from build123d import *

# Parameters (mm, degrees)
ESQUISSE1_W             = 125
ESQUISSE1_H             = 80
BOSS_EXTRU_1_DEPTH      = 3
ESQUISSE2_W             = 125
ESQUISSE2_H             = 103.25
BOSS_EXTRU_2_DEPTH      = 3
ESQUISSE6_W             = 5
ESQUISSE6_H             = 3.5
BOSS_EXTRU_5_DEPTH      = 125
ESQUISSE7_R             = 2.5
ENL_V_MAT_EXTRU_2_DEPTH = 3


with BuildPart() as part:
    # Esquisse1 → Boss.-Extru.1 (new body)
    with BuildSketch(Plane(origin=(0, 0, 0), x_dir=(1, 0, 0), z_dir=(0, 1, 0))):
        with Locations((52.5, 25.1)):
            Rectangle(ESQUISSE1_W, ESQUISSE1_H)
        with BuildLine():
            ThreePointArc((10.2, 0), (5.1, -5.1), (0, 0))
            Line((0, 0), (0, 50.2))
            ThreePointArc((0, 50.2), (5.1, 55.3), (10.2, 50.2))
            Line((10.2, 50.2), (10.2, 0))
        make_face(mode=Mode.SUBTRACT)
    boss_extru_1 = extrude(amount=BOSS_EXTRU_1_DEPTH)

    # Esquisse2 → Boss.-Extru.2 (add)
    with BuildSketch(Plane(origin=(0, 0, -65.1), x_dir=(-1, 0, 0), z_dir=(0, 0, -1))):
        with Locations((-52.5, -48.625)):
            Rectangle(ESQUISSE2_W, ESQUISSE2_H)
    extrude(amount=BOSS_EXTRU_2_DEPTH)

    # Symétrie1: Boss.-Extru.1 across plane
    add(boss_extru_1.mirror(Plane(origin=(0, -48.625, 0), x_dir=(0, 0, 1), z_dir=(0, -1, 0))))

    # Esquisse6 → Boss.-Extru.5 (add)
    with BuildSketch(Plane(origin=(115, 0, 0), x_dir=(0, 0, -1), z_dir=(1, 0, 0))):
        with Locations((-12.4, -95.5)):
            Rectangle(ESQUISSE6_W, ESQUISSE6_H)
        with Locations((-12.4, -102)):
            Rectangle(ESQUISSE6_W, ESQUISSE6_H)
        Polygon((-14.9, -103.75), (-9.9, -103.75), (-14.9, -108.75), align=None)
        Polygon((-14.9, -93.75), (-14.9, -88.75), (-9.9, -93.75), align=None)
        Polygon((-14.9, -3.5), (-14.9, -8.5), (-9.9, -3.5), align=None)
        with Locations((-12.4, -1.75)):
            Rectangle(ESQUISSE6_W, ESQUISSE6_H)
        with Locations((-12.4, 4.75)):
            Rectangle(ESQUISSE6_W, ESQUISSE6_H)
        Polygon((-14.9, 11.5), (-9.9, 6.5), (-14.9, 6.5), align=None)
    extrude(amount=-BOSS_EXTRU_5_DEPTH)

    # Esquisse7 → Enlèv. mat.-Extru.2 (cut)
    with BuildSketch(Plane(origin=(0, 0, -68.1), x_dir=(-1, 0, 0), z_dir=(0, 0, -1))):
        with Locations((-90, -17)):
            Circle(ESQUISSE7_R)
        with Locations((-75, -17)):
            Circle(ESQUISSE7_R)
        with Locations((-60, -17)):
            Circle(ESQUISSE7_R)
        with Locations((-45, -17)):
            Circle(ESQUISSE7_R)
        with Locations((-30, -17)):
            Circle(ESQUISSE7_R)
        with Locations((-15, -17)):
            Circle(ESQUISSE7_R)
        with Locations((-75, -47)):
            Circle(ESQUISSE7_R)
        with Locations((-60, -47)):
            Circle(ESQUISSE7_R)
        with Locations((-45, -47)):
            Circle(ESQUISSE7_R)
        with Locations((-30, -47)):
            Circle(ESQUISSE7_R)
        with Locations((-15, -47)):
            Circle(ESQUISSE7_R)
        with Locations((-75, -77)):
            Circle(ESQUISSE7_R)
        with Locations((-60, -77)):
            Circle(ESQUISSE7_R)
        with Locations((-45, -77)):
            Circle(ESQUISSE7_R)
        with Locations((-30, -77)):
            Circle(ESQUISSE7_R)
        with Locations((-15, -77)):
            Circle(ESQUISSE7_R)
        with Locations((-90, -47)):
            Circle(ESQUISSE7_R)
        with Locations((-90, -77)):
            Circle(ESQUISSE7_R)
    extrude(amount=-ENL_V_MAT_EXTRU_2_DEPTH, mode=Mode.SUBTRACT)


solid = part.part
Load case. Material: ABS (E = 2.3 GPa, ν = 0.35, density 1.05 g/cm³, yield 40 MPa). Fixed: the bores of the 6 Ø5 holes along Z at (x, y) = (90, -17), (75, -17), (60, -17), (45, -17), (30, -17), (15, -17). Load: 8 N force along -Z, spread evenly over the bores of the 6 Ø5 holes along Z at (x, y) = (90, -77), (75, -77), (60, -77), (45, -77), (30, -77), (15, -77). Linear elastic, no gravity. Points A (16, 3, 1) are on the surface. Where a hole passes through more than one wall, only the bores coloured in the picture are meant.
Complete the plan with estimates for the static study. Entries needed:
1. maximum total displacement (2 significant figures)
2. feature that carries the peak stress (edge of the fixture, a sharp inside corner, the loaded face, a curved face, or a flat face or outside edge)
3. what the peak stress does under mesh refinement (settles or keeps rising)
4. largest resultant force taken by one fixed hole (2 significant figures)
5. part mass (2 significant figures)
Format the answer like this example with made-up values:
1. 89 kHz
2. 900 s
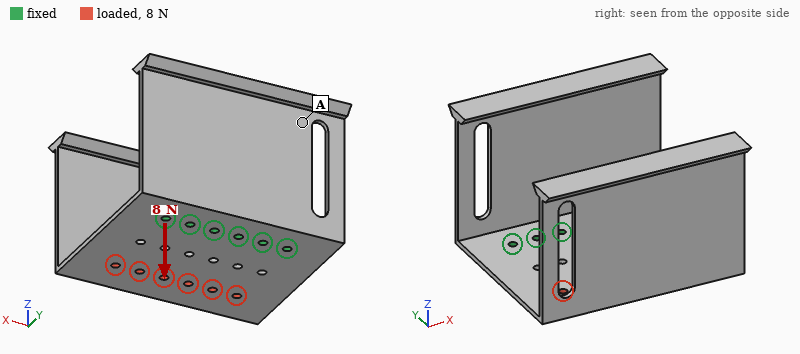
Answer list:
1. 2.3 mm
2. edge of the fixture
3. keeps rising
4. 2.7 N
5. 110 g
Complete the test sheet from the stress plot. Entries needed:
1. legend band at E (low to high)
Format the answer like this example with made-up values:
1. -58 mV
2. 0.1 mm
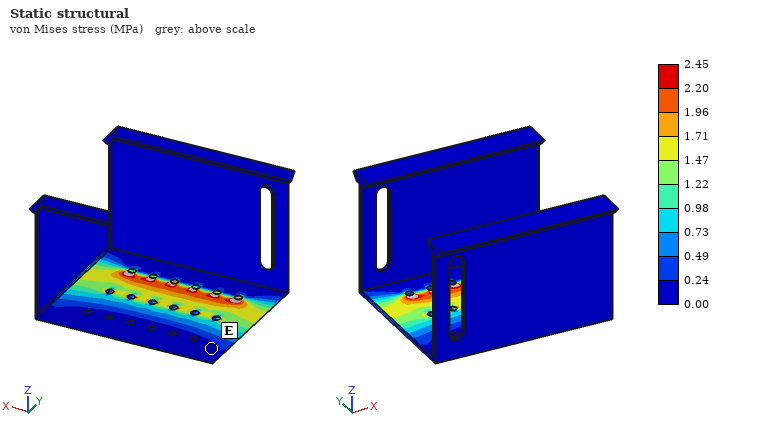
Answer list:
1. 0.00 to 0.24 MPa
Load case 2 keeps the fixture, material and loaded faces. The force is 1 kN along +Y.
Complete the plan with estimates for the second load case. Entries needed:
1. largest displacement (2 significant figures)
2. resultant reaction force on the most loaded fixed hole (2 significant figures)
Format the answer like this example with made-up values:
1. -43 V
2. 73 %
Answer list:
1. 0.12 mm
2. 240 N
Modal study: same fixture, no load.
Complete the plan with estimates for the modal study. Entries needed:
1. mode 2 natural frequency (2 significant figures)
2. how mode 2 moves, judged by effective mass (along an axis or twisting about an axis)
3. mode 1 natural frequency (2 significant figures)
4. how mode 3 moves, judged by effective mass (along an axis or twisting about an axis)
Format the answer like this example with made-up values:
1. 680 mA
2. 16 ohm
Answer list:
1. 55 Hz
2. along X
3. 31 Hz
4. along Y
